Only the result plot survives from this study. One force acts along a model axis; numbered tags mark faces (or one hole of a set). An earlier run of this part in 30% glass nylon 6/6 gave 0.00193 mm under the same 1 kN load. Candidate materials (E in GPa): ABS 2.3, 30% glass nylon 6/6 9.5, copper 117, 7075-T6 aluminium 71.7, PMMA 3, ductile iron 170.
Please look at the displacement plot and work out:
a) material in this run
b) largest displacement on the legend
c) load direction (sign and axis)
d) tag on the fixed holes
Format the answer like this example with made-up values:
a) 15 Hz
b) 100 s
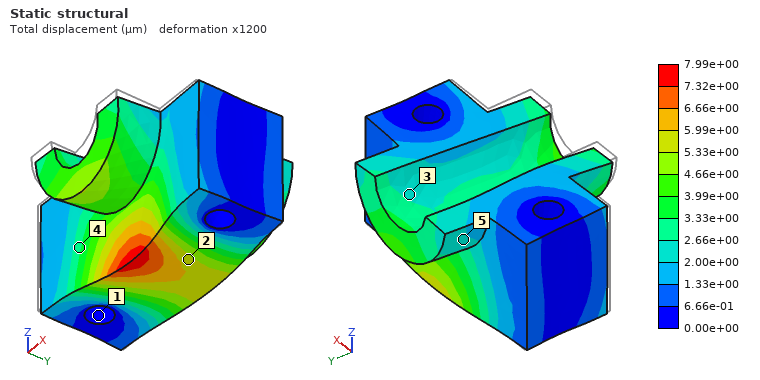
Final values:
a) ABS
b) 7.99e+00 µm
c) +Y
d) 1
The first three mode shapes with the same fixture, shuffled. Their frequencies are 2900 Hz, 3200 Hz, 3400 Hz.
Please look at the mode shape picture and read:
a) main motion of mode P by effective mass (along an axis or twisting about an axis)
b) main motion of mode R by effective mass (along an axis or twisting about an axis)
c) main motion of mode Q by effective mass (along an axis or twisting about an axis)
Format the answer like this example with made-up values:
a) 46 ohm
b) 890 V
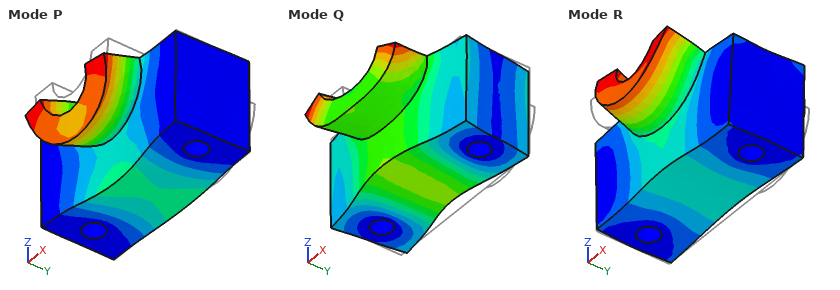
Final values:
a) twisting about X
b) along Z
c) along Y
